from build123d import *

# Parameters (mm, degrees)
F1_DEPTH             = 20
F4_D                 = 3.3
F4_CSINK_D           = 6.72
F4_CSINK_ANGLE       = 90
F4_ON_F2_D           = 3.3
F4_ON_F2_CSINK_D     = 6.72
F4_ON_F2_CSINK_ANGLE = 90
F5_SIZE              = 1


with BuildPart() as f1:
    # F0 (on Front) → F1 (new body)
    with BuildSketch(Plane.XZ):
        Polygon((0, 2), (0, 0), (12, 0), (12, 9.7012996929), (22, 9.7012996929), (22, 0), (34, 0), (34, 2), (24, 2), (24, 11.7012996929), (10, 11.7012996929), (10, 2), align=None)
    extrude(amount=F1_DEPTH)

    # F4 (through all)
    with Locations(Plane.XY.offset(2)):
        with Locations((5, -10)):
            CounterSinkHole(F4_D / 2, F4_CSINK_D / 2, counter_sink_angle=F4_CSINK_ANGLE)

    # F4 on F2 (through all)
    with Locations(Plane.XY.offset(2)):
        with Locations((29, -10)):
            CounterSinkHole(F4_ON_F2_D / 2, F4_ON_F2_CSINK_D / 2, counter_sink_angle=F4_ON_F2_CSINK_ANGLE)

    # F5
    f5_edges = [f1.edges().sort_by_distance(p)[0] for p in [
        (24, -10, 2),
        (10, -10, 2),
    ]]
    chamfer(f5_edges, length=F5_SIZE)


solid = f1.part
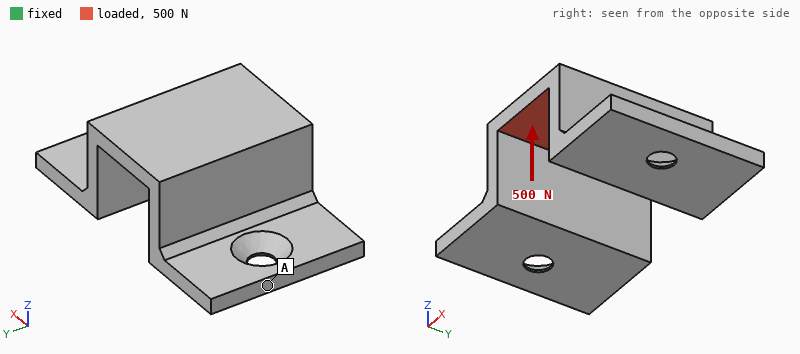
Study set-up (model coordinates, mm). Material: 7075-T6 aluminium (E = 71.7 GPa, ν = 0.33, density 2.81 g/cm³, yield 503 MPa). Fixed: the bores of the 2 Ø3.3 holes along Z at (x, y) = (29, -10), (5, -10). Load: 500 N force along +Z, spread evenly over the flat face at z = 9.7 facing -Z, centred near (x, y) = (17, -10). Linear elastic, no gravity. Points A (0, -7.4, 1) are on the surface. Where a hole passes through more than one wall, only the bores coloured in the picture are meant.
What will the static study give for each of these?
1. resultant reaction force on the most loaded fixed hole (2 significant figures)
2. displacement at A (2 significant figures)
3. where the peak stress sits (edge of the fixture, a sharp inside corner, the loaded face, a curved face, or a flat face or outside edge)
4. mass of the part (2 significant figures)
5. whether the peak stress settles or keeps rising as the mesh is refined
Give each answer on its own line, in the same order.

300 N
6.2 µm
edge of the fixture
5.8 g
keeps rising
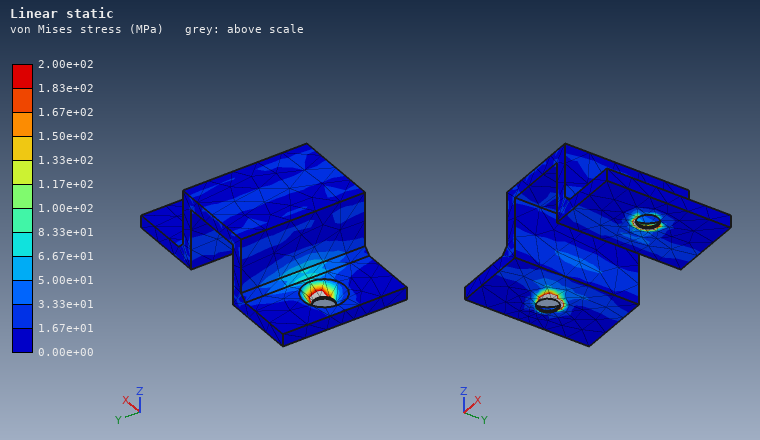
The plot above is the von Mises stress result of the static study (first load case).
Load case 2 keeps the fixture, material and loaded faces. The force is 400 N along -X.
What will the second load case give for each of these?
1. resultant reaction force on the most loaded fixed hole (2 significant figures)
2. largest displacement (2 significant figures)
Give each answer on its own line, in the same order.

260 N
32 µm
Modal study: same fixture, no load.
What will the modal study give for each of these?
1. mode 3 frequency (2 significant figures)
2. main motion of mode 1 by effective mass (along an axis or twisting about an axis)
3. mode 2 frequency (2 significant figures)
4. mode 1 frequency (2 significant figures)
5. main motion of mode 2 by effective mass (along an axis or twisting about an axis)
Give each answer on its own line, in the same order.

12 kHz
along Y
11 kHz
3100 Hz
along X
